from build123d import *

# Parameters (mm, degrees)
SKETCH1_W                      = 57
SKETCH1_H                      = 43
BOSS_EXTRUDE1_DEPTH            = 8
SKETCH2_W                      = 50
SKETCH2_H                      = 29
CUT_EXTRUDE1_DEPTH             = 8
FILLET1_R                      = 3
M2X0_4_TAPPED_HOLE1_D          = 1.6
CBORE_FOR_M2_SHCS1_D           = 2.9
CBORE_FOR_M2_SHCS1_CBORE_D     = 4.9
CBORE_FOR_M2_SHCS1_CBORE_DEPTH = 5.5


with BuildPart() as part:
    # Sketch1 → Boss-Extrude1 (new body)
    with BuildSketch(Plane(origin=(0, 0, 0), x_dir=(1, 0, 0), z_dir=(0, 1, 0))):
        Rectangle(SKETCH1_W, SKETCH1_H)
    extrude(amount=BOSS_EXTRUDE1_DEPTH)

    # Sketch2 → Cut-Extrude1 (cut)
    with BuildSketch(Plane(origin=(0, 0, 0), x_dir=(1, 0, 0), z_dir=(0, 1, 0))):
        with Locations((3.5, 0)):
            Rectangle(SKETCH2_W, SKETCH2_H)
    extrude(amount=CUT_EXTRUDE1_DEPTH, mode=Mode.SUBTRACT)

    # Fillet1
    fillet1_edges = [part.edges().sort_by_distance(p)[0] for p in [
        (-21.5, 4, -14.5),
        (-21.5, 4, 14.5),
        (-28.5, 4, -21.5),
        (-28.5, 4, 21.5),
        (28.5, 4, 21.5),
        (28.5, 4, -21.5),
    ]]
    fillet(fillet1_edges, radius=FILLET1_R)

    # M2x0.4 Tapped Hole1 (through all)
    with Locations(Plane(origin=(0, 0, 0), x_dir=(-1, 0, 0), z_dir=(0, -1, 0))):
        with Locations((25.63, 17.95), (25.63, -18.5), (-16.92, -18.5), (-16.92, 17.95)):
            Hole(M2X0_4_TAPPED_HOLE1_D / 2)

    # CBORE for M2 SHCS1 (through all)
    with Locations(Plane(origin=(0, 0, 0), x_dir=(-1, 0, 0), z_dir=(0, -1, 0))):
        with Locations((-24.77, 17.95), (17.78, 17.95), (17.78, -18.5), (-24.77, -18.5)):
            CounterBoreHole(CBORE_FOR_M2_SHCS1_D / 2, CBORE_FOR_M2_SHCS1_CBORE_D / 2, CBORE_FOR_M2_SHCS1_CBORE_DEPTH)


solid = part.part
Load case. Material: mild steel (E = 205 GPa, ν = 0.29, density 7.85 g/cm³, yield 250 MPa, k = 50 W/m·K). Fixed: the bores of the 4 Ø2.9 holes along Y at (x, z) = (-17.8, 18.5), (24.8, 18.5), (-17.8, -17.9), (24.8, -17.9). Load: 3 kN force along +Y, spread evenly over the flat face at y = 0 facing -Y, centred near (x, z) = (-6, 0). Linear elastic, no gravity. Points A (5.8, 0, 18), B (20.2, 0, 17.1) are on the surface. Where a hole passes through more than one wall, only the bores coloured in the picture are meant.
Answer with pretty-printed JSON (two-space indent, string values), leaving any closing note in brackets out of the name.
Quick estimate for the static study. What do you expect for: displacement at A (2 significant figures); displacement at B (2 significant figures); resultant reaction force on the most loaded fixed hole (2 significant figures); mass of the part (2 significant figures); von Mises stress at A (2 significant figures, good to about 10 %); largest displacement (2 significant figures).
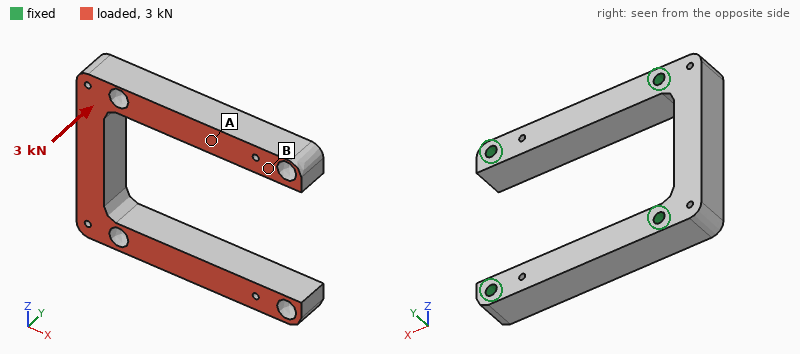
{
  "displacement at A": "6.6 µm",
  "displacement at B": "3.3 µm",
  "resultant reaction force on the most loaded fixed hole": "1.1 kN",
  "mass of the part": "58 g",
  "von Mises stress at A": "32 MPa",
  "largest displacement": "10 µm"
}
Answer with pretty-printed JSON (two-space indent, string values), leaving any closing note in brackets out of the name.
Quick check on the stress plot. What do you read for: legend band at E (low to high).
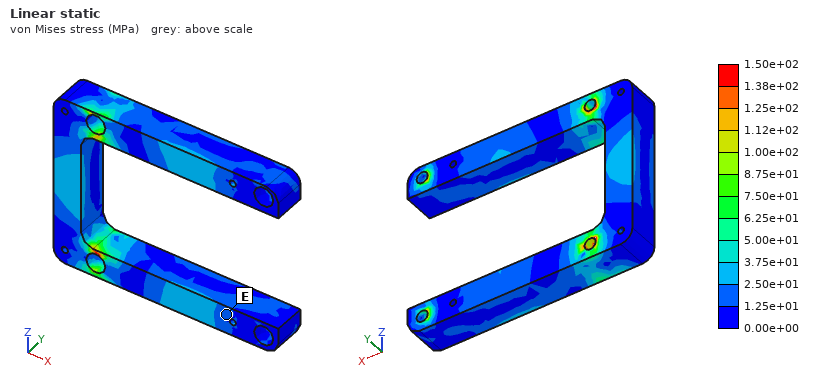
{
  "legend band at E": "1.25e+01 to 2.50e+01 MPa"
}
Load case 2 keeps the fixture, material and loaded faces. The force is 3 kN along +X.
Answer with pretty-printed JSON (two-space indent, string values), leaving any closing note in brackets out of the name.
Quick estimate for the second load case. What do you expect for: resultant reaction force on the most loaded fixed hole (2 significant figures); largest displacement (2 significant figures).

{
  "resultant reaction force on the most loaded fixed hole": "840 N",
  "largest displacement": "14 µm"
}
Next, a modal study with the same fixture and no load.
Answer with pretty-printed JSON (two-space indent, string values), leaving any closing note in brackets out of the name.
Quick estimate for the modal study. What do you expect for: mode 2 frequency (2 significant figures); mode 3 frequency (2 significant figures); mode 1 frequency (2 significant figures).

{
  "mode 2 frequency": "13 kHz",
  "mode 3 frequency": "13 kHz",
  "mode 1 frequency": "11 kHz"
}
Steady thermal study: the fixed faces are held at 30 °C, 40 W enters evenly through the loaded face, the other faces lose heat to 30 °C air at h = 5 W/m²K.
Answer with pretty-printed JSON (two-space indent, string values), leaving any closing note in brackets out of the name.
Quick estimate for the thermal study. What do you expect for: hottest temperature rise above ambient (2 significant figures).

{
  "hottest temperature rise above ambient": "43 K"
}
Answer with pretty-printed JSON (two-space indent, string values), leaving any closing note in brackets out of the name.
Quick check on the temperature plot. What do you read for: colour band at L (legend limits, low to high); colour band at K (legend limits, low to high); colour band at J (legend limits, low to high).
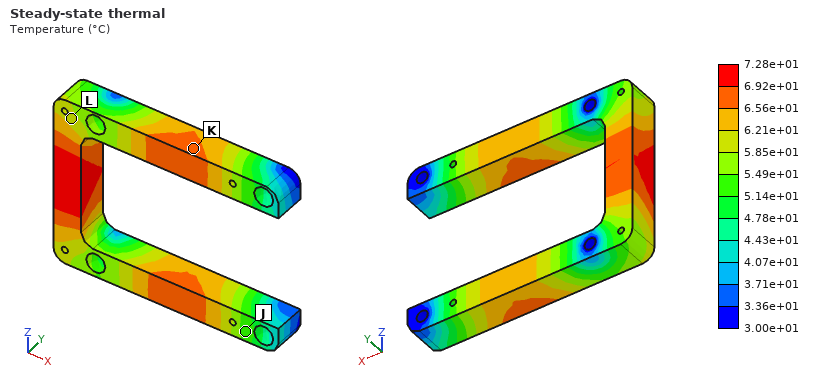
{
  "colour band at L": "5.85e+01 to 6.21e+01 °C",
  "colour band at K": "6.56e+01 to 6.92e+01 °C",
  "colour band at J": "5.14e+01 to 5.49e+01 °C"
}
